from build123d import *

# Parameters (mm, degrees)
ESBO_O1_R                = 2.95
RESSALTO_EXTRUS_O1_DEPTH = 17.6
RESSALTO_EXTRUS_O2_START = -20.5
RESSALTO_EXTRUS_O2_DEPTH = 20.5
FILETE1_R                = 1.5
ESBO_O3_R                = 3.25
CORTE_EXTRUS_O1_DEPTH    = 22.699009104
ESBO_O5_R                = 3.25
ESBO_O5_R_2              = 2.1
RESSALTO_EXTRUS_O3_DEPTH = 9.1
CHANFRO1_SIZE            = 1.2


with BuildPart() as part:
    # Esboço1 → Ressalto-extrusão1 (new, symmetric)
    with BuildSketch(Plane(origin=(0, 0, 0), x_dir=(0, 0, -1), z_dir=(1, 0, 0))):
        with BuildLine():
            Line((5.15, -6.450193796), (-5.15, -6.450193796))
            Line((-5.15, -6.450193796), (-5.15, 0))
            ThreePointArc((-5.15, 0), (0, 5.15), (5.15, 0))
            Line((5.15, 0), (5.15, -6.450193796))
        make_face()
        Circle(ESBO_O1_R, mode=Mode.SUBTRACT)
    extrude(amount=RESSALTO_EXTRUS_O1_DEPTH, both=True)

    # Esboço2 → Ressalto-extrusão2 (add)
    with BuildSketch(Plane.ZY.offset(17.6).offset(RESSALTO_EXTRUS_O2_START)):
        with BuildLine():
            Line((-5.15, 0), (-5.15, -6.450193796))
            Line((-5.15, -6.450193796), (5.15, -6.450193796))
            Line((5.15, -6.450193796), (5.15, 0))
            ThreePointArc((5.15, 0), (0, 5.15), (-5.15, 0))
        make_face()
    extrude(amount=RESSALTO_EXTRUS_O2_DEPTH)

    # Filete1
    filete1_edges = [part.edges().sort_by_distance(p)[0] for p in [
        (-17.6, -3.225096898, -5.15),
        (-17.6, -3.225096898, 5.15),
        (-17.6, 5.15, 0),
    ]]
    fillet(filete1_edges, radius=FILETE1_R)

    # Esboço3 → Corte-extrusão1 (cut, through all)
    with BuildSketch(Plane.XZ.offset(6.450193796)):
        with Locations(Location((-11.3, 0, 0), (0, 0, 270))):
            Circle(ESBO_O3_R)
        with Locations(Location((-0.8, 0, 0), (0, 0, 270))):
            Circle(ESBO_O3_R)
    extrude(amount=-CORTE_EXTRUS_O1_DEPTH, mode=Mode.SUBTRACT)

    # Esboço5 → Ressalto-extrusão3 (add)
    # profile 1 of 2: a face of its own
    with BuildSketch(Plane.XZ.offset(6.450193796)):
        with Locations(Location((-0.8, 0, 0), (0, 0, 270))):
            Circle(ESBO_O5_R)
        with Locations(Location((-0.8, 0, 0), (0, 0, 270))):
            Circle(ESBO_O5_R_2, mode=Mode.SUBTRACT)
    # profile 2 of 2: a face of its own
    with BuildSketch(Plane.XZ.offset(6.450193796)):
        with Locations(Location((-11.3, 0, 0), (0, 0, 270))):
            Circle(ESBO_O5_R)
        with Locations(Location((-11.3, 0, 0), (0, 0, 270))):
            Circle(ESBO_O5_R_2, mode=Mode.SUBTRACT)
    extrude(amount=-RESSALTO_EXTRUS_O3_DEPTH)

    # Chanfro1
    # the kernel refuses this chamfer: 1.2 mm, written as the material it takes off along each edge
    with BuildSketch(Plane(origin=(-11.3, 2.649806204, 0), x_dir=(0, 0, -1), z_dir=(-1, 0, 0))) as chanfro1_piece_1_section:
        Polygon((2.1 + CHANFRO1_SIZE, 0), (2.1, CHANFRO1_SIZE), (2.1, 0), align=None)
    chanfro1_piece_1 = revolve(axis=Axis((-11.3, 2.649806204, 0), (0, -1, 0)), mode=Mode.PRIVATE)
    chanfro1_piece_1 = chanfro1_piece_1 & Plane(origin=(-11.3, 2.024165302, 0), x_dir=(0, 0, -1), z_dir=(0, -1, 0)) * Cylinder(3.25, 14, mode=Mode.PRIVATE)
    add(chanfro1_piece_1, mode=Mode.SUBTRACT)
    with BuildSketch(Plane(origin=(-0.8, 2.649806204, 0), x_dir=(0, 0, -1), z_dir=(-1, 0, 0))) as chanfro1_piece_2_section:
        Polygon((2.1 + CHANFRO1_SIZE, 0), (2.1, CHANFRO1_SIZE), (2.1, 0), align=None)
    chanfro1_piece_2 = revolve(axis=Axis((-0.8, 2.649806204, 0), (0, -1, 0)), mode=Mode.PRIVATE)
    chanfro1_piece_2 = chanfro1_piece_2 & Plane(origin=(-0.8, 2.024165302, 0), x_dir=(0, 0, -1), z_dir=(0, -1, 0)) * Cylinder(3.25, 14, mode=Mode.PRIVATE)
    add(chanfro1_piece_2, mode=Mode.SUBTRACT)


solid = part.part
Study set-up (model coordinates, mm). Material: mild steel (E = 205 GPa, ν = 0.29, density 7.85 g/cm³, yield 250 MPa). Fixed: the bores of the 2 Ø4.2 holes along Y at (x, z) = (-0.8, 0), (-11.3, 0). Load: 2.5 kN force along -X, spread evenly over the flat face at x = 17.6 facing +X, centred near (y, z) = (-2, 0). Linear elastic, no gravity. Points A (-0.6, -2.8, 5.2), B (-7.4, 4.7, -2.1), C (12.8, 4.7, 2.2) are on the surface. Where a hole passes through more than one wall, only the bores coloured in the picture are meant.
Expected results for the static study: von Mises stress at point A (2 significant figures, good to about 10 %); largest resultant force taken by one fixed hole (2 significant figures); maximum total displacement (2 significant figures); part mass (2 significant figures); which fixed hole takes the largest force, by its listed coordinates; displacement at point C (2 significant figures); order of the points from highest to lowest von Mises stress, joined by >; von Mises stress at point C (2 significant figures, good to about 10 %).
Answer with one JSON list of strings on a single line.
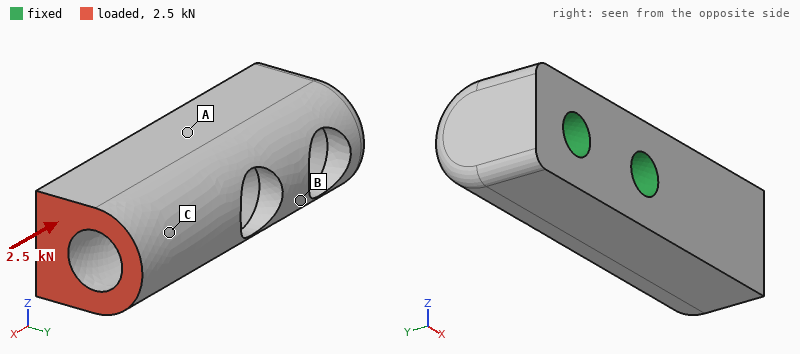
["17 MPa", "2.2 kN", "4.8 µm", "23 g", "(-0.8, 0)", "3.7 µm", "C > A > B", "31 MPa"]
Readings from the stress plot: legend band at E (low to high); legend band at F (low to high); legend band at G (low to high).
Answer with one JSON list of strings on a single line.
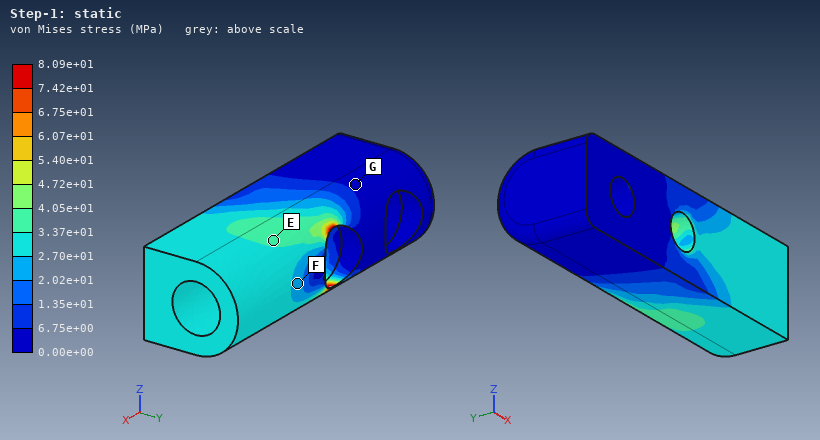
["3.37e+01 to 4.05e+01 MPa", "2.02e+01 to 2.70e+01 MPa", "0.00e+00 to 6.75e+00 MPa"]
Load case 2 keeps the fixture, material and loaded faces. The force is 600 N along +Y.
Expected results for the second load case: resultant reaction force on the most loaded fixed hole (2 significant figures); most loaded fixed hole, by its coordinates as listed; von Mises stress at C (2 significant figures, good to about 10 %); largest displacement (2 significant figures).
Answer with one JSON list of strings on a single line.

["790 N", "(-0.8, 0)", "22 MPa", "14 µm"]
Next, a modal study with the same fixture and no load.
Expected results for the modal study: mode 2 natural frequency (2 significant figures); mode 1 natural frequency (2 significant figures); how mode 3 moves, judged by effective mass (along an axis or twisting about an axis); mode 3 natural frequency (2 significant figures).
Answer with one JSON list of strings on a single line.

["19 kHz", "19 kHz", "twisting about X", "39 kHz"]
